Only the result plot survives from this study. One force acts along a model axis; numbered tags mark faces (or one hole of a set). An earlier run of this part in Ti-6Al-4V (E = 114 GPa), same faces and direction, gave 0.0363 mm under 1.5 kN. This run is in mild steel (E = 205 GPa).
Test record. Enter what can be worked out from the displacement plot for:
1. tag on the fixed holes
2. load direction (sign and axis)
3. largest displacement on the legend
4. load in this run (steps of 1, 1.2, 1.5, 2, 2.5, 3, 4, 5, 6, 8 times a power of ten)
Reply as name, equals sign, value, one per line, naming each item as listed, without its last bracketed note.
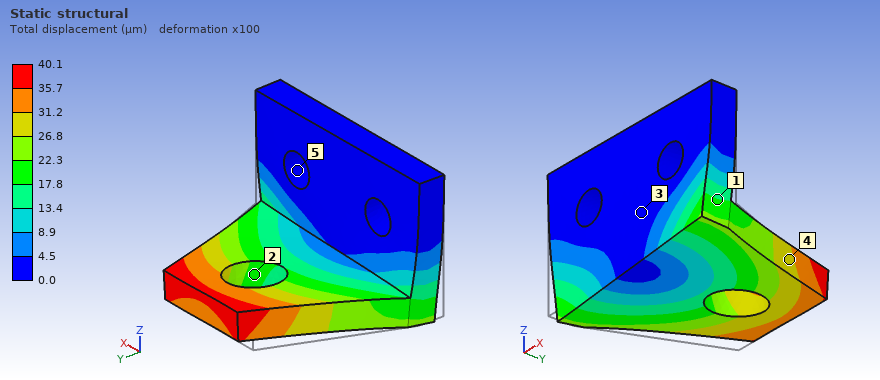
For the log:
tag on the fixed holes = 5
load direction = +X
largest displacement on the legend = 40.1 µm
load in this run = 3 kN
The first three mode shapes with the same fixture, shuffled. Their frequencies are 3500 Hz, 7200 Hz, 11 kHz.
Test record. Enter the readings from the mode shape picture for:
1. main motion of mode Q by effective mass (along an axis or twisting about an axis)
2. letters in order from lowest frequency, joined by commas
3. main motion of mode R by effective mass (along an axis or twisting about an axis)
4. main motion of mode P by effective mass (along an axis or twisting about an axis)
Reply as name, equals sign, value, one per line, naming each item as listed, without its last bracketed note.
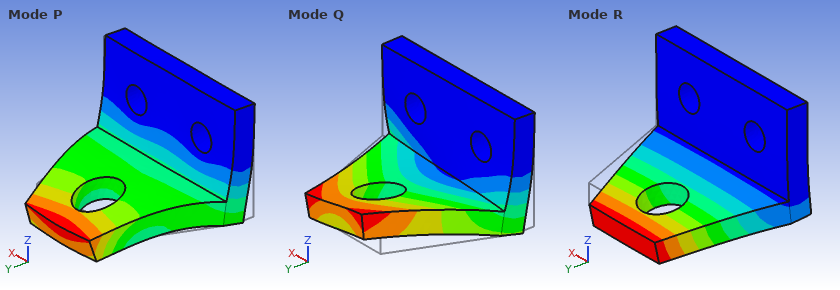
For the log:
main motion of mode Q by effective mass = along X
letters in order from lowest frequency, joined by commas = R, Q, P
main motion of mode R by effective mass = along Z
main motion of mode P by effective mass = along Y
